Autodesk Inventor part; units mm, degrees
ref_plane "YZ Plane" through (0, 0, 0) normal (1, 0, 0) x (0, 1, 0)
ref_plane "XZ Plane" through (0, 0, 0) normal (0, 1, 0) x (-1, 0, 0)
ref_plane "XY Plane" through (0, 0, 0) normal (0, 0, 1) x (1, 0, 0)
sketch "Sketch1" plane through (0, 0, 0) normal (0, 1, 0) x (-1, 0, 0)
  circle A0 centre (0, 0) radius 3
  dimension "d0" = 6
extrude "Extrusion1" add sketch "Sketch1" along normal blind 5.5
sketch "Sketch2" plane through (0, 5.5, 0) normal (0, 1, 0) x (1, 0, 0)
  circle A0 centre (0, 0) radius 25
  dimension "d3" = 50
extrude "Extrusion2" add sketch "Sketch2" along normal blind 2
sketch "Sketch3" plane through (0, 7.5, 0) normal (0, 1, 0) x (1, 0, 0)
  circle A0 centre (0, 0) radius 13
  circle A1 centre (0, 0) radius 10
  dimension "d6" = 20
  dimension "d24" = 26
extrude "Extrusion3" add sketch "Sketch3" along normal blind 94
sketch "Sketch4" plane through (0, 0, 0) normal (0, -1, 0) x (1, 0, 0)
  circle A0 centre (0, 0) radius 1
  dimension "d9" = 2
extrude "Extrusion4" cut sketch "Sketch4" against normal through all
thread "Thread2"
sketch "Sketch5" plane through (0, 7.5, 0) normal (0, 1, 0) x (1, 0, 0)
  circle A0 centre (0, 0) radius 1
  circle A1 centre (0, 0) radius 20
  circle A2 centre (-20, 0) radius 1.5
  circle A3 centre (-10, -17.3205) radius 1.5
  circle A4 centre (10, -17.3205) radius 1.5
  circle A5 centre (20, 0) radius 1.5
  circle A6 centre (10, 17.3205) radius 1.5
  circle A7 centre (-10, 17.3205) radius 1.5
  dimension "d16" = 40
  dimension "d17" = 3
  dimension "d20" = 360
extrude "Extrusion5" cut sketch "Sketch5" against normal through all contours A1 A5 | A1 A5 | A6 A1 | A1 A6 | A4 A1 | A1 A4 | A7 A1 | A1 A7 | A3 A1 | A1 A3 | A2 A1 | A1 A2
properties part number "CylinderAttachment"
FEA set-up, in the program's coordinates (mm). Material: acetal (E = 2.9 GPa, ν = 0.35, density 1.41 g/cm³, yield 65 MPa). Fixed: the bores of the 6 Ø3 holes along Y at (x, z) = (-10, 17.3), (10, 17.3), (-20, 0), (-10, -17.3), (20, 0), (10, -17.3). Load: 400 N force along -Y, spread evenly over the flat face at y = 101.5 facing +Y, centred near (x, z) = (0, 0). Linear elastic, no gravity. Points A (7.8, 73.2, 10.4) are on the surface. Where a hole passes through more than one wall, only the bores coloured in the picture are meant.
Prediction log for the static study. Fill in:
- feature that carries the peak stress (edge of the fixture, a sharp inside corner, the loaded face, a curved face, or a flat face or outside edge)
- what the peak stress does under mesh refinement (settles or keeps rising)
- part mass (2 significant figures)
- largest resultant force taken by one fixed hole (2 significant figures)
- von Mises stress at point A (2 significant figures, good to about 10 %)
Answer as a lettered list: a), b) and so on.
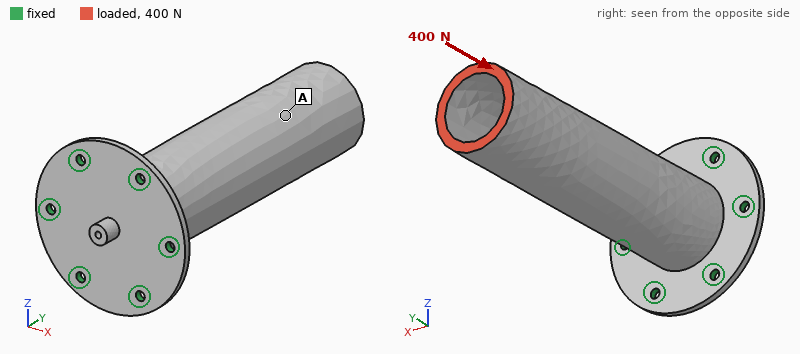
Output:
a) edge of the fixture
b) keeps rising
c) 34 g
d) 72 N
e) 1.8 MPa
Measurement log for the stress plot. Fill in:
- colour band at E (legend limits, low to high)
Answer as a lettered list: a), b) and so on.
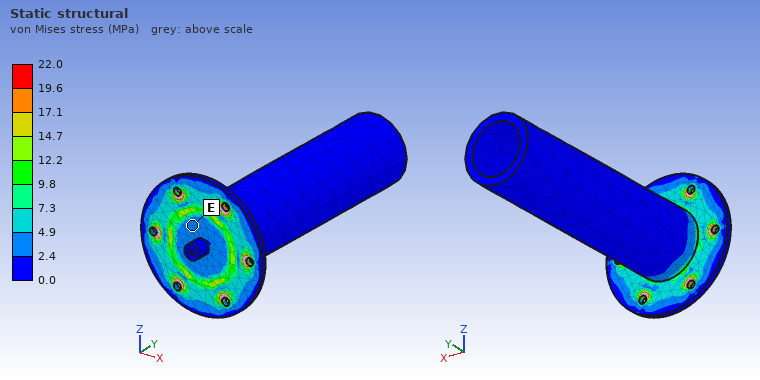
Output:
a) 2.4 to 4.9 MPa
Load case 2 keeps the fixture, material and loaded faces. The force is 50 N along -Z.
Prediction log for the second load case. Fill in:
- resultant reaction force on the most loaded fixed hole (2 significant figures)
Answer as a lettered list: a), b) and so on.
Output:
a) 84 N
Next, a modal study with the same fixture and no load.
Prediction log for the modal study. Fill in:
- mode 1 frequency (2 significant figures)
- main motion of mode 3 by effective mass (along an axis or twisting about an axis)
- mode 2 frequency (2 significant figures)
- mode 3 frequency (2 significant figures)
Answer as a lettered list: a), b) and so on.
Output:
a) 310 Hz
b) along Y
c) 310 Hz
d) 1500 Hz
